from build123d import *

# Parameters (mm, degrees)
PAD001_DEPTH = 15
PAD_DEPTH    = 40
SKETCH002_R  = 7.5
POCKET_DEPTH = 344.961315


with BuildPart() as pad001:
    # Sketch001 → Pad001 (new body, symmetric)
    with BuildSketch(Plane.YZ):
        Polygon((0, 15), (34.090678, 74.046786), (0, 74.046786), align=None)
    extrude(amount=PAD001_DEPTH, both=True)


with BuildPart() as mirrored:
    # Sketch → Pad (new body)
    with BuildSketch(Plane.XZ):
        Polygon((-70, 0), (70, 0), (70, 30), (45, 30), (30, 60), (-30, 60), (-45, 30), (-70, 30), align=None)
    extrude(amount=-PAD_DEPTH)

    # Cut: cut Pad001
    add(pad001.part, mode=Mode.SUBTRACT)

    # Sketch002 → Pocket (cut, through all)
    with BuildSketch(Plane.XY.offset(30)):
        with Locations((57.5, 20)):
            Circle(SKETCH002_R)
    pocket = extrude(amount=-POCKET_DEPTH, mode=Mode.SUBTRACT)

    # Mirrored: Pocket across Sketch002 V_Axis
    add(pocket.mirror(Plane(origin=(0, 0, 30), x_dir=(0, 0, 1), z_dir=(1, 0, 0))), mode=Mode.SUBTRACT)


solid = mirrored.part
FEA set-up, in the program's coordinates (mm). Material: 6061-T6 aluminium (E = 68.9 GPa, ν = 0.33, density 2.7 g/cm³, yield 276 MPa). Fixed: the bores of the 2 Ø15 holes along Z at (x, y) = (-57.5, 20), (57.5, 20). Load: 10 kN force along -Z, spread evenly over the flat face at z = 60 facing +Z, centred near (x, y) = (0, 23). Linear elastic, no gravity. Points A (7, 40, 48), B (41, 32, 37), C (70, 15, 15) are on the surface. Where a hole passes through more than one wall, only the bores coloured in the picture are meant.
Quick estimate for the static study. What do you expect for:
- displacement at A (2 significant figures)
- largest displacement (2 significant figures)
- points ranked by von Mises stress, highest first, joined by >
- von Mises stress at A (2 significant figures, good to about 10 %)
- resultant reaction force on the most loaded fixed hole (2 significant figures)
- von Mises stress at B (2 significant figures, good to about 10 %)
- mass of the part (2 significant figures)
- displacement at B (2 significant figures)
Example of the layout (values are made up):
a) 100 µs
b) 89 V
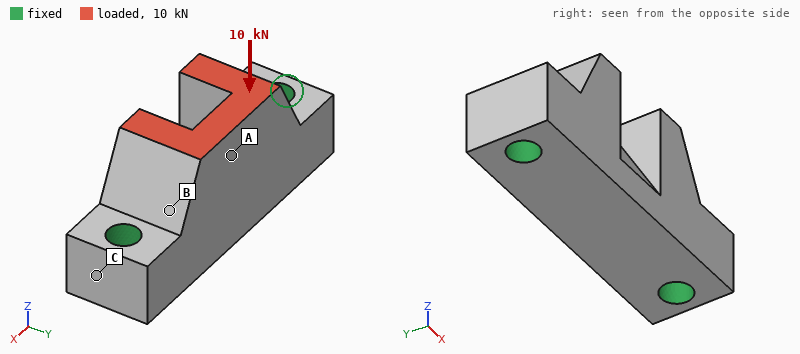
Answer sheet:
a) 12 µm
b) 14 µm
c) B > A > C
d) 5.3 MPa
e) 5.4 kN
f) 9.3 MPa
g) 620 g
h) 5.3 µm
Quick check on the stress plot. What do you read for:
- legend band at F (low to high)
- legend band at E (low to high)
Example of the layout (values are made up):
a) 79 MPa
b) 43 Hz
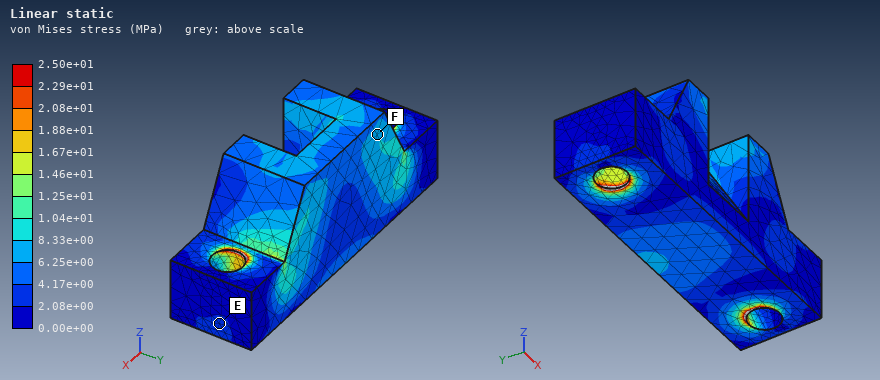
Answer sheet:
a) 6.25e+00 to 8.33e+00 MPa
b) 2.08e+00 to 4.17e+00 MPa
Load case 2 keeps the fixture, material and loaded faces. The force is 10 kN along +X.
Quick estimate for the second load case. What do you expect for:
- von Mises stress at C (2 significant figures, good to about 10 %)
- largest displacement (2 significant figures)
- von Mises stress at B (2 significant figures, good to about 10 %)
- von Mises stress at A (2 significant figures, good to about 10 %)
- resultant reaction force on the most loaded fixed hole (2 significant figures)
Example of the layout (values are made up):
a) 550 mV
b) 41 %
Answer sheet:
a) 2.1 MPa
b) 18 µm
c) 13 MPa
d) 8.6 MPa
e) 6.6 kN
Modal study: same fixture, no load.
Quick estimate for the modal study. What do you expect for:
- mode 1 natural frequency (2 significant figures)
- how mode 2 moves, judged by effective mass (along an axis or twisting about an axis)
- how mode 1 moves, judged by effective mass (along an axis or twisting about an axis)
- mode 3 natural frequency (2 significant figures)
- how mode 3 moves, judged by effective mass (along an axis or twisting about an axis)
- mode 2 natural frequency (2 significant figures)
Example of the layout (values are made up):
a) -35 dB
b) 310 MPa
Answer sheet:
a) 5800 Hz
b) along Z
c) along Y
d) 9700 Hz
e) along Y
f) 8900 Hz
